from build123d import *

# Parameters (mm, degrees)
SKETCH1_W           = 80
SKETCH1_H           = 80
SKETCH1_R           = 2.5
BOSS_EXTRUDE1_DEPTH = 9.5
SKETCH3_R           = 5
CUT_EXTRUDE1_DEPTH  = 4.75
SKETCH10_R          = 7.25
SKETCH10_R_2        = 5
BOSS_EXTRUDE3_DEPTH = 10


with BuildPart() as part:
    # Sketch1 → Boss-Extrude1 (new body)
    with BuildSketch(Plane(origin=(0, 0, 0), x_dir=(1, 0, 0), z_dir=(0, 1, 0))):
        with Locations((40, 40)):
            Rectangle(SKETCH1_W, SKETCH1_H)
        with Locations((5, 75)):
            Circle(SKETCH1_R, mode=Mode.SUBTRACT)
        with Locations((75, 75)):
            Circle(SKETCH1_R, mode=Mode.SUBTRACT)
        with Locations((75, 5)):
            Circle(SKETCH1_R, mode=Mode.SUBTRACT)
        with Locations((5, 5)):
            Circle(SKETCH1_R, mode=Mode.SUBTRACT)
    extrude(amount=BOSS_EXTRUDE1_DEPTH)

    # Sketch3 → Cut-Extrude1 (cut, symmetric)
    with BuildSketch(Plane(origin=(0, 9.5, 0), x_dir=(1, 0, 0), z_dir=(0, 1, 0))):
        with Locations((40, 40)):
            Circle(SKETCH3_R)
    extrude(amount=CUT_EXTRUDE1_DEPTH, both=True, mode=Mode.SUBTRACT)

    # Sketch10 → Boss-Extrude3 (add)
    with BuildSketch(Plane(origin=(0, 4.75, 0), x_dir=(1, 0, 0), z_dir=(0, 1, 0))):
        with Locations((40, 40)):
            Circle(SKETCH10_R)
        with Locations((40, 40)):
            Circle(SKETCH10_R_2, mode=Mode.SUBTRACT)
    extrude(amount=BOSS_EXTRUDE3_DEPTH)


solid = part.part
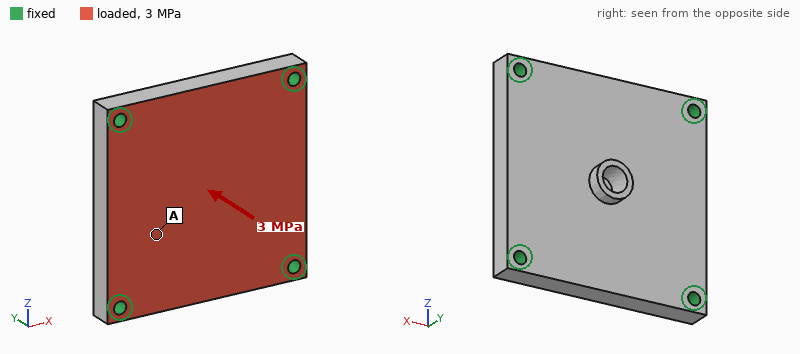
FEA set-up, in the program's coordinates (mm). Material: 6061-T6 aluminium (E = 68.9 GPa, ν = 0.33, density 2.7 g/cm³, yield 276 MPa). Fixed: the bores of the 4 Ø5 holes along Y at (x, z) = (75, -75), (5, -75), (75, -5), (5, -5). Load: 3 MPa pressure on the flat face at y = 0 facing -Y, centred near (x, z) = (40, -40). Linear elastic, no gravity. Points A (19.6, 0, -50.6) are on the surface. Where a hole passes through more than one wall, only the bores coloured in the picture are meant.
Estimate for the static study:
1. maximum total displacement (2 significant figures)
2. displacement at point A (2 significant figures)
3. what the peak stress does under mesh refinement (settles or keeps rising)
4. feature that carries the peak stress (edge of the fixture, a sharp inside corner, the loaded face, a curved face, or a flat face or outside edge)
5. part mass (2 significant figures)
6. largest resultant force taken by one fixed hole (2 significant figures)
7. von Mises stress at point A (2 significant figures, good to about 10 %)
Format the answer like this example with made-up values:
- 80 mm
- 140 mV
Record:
- 0.13 mm
- 0.095 mm
- keeps rising
- edge of the fixture
- 160 g
- 4.7 kN
- 42 MPa
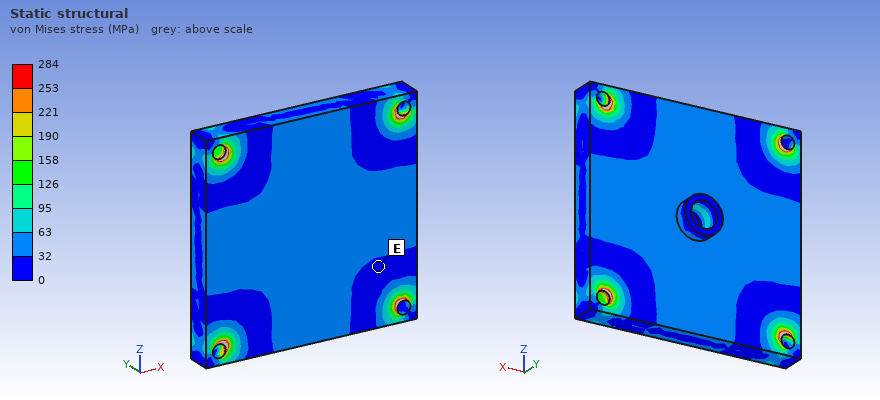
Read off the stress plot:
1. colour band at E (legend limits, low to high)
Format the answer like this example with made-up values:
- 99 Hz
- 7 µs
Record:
- 0 to 32 MPa
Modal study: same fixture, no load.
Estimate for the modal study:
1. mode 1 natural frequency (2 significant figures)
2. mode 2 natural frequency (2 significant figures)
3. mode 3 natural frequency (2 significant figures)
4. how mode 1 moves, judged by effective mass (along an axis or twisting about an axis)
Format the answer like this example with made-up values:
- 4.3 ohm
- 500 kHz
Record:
- 5800 Hz
- 9700 Hz
- 9700 Hz
- along Y
